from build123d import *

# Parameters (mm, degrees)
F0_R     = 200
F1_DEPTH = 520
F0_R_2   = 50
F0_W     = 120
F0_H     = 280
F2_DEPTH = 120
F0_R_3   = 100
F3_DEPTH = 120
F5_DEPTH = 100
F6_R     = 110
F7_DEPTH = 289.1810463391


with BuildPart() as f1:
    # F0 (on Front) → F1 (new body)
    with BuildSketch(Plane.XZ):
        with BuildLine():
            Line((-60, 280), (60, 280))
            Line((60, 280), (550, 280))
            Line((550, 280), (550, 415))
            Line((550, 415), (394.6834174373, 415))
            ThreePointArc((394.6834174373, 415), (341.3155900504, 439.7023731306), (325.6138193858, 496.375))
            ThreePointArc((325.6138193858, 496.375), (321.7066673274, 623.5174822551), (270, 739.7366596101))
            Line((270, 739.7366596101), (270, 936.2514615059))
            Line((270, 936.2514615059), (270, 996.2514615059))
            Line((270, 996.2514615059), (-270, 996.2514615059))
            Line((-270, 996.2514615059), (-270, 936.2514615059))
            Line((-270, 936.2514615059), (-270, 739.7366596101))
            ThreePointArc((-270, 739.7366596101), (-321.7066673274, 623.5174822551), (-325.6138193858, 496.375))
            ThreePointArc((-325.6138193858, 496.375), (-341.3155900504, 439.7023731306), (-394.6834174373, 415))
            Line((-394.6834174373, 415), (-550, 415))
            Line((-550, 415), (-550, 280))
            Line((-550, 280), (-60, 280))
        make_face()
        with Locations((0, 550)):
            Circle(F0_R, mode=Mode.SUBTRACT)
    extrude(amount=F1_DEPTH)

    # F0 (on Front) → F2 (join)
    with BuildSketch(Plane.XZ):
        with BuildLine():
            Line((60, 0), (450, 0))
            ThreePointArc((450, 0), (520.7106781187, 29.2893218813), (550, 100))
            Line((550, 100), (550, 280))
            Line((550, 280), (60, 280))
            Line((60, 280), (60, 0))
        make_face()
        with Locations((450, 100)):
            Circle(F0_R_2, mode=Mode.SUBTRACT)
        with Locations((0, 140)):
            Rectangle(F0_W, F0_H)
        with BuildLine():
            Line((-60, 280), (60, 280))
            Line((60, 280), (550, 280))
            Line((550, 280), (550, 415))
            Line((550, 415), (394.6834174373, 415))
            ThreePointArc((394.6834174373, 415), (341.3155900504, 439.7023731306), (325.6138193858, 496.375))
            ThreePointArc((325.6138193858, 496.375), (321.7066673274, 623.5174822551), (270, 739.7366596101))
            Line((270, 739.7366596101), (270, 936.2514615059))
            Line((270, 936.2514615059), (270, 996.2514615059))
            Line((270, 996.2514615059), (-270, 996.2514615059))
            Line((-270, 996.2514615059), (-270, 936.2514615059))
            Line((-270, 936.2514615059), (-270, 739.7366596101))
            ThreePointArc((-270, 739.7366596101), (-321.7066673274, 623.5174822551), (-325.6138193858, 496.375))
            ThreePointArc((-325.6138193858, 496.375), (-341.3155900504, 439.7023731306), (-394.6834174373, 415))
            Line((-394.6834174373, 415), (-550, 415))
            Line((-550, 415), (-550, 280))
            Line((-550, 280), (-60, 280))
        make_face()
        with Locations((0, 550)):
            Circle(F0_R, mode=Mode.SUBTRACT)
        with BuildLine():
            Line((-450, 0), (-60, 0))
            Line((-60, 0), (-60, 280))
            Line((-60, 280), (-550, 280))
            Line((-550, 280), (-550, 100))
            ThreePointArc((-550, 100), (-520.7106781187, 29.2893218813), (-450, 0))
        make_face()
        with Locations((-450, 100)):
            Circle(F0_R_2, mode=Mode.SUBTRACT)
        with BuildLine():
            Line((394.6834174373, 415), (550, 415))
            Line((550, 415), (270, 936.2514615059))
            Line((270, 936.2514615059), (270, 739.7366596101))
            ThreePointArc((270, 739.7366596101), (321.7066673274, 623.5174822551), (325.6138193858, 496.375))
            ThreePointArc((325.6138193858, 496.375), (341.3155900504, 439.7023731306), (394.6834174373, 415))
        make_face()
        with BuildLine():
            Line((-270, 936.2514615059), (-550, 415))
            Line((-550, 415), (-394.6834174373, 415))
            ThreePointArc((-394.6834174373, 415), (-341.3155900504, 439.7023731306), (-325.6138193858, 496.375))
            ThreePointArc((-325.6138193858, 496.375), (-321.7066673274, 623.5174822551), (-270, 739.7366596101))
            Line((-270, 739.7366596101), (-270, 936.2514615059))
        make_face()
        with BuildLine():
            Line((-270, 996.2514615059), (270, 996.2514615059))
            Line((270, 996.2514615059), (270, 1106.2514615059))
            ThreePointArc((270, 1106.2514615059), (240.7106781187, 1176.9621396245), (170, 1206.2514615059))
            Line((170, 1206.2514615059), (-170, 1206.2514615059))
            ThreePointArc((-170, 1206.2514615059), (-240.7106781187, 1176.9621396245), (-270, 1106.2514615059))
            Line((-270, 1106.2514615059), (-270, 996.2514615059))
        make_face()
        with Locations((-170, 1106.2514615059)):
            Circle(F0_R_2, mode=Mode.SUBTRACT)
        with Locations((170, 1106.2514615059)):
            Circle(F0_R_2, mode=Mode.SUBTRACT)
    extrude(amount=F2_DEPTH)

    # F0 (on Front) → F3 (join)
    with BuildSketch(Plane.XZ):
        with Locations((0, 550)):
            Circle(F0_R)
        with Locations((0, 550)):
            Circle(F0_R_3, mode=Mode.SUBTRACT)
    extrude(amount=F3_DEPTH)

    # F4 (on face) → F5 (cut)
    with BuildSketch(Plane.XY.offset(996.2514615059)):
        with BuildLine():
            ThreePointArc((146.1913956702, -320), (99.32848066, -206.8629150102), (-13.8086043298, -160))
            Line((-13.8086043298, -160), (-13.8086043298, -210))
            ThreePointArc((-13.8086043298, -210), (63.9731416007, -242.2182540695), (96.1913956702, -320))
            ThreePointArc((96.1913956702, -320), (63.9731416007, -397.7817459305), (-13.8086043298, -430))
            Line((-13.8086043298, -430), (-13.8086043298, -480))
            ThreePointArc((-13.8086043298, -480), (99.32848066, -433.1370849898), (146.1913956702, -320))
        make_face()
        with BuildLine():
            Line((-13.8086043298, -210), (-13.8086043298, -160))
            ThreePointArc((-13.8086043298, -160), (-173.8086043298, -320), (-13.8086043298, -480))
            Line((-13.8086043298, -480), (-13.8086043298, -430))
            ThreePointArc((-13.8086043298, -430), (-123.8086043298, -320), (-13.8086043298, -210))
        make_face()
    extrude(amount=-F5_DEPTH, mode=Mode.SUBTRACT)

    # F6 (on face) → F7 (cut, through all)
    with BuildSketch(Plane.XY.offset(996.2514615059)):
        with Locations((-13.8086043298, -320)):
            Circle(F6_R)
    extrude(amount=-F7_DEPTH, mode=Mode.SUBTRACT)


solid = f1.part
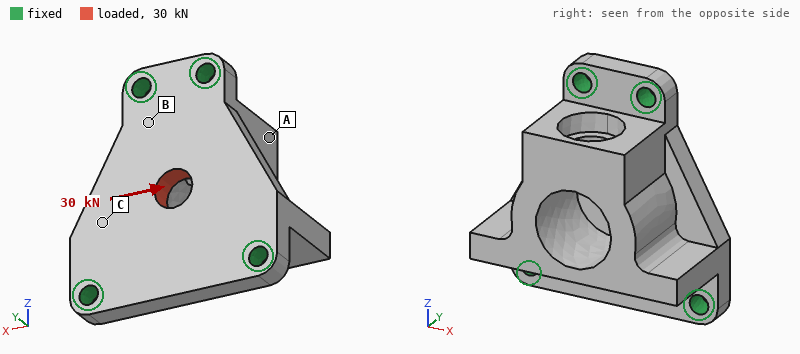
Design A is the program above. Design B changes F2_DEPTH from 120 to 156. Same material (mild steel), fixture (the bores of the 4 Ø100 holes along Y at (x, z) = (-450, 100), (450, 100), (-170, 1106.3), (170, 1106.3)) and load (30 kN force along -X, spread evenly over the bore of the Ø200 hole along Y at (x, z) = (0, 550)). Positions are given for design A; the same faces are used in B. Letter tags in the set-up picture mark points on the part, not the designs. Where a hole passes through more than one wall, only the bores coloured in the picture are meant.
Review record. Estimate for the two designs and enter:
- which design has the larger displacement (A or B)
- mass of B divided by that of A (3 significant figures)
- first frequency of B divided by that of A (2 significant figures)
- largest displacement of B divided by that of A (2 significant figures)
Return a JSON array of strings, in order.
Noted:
["A", "1.07", "1.2", "0.89"]
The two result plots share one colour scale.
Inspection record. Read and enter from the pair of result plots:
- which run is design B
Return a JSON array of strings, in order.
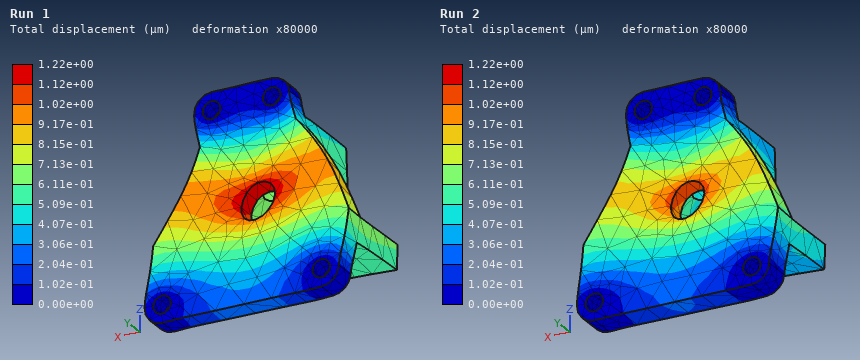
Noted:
["Run 2"]
